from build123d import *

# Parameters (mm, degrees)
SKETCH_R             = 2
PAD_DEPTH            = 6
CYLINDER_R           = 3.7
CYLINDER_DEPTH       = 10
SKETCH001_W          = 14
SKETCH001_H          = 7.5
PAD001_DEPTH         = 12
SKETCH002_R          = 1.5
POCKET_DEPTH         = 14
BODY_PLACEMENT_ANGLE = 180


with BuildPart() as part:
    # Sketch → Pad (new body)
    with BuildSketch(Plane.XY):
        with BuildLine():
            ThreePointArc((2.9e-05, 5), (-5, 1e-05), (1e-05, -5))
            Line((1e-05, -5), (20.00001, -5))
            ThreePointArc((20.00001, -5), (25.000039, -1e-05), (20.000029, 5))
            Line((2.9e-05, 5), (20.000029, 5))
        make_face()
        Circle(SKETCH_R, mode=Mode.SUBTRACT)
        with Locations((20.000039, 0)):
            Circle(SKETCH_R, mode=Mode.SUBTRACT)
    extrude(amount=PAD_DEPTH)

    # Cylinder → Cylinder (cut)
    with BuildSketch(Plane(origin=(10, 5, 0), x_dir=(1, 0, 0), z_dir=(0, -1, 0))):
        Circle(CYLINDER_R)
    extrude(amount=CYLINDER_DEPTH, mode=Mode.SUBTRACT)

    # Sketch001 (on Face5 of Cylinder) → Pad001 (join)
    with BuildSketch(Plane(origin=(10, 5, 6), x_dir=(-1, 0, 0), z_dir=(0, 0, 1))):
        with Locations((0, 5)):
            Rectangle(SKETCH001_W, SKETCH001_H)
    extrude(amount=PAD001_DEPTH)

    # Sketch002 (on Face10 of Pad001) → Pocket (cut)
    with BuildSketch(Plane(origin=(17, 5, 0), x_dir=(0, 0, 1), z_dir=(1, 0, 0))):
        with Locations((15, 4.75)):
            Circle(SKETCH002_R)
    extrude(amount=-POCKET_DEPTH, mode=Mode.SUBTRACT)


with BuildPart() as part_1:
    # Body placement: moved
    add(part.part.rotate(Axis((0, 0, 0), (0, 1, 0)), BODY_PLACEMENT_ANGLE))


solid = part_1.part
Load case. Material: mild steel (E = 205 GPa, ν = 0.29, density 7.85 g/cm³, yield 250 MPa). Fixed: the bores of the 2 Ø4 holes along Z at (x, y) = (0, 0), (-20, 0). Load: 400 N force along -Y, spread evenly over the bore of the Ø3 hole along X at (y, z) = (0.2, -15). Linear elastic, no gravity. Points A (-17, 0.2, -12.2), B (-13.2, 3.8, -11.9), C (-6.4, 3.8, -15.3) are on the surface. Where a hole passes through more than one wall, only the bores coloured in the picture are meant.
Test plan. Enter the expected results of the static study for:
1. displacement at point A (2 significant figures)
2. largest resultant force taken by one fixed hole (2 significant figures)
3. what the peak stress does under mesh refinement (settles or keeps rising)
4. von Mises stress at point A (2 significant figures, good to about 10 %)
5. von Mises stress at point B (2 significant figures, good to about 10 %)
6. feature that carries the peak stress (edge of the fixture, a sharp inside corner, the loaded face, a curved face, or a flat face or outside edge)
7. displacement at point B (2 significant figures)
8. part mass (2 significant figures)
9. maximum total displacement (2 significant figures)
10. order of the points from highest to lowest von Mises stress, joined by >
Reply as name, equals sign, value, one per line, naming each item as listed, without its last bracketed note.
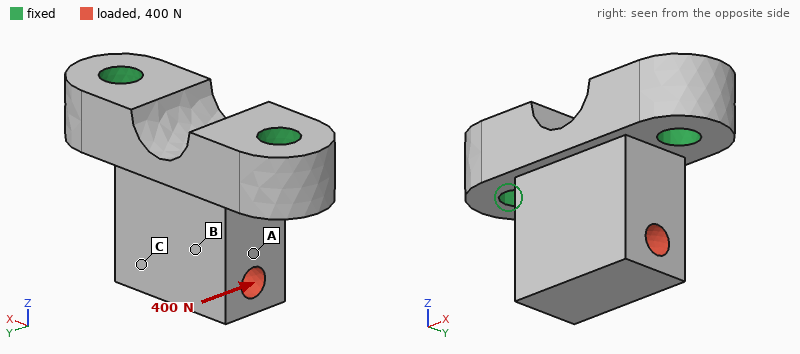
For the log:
displacement at point A = 3.7 µm
largest resultant force taken by one fixed hole = 200 N
what the peak stress does under mesh refinement = keeps rising
von Mises stress at point A = 18 MPa
von Mises stress at point B = 12 MPa
feature that carries the peak stress = edge of the fixture
displacement at point B = 4.0 µm
part mass = 19 g
maximum total displacement = 7.1 µm
order of the points from highest to lowest von Mises stress, joined by > = A > B > C
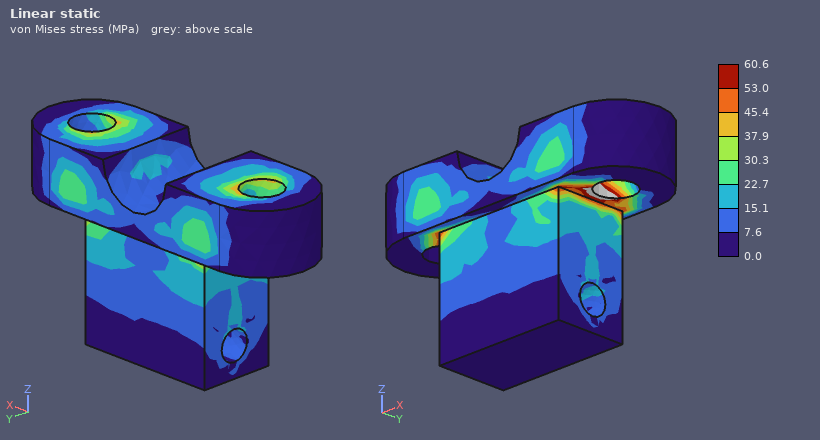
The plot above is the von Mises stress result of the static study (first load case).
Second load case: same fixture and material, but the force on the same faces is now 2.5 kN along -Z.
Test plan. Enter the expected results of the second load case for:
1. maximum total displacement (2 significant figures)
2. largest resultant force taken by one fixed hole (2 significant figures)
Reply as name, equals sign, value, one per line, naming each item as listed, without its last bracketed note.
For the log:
maximum total displacement = 3.7 µm
largest resultant force taken by one fixed hole = 1.4 kN
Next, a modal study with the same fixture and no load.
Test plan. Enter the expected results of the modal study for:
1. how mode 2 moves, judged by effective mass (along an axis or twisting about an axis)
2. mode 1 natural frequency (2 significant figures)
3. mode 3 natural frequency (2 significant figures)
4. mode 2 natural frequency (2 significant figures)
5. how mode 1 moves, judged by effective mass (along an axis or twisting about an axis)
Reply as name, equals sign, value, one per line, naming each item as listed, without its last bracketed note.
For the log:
how mode 2 moves, judged by effective mass = along X
mode 1 natural frequency = 18 kHz
mode 3 natural frequency = 47 kHz
mode 2 natural frequency = 36 kHz
how mode 1 moves, judged by effective mass = along Y
